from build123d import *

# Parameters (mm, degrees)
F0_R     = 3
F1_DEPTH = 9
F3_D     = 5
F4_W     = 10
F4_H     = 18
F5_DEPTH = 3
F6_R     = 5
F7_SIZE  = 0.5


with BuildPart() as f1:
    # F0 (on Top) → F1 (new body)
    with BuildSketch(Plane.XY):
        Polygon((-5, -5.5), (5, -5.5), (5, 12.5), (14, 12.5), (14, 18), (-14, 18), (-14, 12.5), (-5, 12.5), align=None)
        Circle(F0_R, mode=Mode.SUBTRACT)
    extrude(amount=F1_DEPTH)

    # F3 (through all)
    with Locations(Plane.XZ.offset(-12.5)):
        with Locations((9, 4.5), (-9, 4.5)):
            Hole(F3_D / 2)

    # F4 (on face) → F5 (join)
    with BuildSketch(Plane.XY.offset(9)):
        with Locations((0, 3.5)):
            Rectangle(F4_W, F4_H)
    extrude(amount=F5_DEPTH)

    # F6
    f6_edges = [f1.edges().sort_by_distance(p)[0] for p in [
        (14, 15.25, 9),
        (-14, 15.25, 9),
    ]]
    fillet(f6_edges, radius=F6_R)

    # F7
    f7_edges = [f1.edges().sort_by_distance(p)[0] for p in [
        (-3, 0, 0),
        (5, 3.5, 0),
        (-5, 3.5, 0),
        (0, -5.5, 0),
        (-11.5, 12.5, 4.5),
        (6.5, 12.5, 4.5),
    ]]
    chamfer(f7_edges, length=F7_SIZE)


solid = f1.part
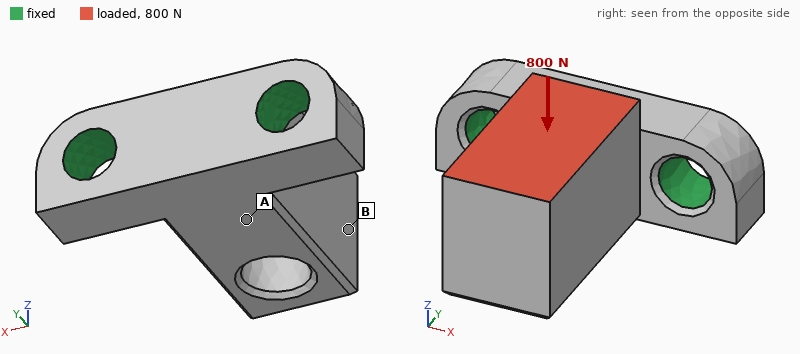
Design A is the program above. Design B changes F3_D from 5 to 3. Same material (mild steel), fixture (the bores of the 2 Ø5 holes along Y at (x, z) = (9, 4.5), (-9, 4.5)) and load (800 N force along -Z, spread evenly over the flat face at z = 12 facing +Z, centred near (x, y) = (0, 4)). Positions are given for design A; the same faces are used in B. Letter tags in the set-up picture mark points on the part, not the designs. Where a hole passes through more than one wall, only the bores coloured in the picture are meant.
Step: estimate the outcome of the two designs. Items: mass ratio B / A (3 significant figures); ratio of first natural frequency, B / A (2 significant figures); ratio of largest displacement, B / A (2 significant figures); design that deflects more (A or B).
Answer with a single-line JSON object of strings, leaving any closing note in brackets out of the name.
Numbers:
{"mass ratio B / A": "1.05", "ratio of first natural frequency, B / A": "0.87", "ratio of largest displacement, B / A": "1.3", "design that deflects more": "B"}
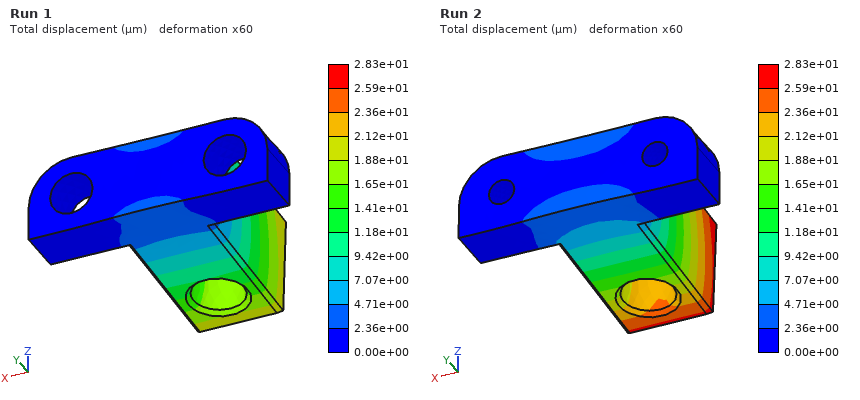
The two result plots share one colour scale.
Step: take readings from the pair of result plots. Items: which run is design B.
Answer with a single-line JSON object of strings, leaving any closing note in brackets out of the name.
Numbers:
{"which run is design B": "Run 2"}
